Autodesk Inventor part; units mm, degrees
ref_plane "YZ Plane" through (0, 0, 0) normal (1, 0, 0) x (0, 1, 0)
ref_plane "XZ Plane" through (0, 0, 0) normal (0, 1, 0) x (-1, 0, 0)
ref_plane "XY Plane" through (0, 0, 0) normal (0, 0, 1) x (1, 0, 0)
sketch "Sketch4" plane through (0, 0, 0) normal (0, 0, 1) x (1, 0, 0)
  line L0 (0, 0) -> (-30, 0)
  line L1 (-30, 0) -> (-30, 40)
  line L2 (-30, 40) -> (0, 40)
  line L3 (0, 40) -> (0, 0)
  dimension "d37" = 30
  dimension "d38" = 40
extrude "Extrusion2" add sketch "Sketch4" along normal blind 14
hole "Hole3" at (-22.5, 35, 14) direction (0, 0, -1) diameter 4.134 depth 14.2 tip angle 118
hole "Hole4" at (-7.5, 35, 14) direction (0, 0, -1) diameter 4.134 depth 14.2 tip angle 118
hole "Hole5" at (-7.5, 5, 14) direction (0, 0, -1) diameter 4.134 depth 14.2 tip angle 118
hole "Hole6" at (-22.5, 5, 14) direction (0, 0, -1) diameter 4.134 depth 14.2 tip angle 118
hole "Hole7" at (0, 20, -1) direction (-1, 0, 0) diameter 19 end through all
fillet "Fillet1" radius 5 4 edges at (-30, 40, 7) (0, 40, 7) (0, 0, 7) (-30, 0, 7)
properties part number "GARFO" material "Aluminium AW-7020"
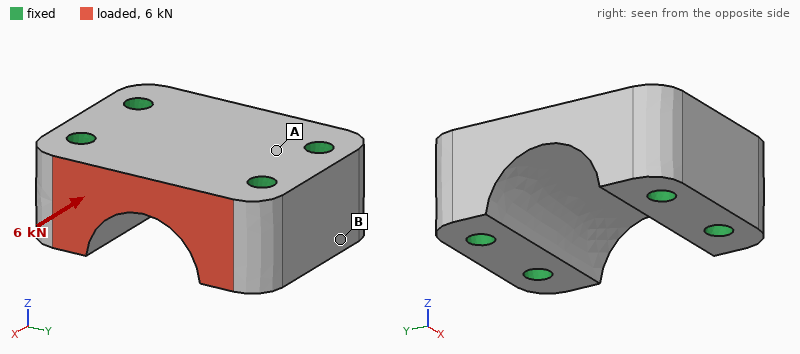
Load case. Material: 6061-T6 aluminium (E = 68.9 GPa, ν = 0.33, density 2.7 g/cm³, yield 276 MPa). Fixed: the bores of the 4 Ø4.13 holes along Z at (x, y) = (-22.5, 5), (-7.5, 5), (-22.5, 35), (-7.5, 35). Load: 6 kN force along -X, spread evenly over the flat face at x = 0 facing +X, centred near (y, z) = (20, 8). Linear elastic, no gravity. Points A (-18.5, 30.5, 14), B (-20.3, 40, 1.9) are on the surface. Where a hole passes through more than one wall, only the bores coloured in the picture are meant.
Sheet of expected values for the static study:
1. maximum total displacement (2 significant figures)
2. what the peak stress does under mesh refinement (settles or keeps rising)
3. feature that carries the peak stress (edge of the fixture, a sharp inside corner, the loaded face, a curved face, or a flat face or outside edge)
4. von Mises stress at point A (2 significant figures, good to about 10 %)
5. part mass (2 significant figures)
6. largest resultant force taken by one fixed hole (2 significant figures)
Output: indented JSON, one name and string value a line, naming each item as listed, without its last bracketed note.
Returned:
{
  "maximum total displacement": "7.0 µm",
  "what the peak stress does under mesh refinement": "keeps rising",
  "feature that carries the peak stress": "edge of the fixture",
  "von Mises stress at point A": "14 MPa",
  "part mass": "33 g",
  "largest resultant force taken by one fixed hole": "2.2 kN"
}
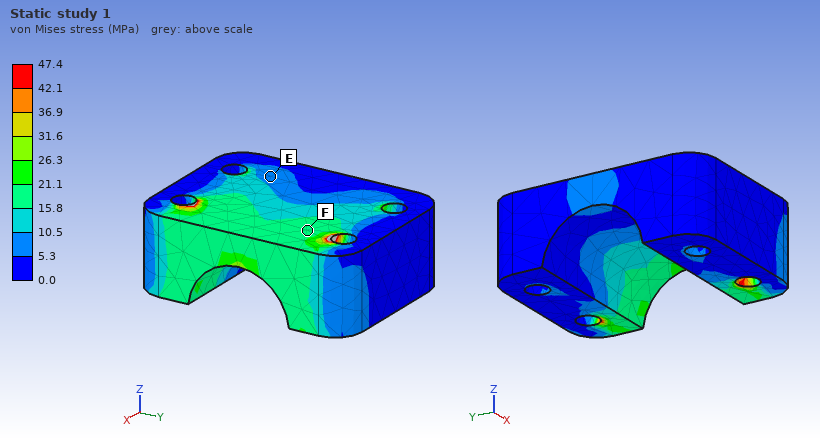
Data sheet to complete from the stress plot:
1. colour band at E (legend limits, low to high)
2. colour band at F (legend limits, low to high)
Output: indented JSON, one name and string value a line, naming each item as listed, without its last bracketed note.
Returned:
{
  "colour band at E": "5.3 to 10.5 MPa",
  "colour band at F": "15.8 to 21.1 MPa"
}
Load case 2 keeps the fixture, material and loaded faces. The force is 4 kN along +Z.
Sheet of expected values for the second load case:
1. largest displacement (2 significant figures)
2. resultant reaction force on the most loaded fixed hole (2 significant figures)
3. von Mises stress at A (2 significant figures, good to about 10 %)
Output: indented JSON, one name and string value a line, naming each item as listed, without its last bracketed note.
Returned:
{
  "largest displacement": "16 µm",
  "resultant reaction force on the most loaded fixed hole": "2.1 kN",
  "von Mises stress at A": "7.5 MPa"
}
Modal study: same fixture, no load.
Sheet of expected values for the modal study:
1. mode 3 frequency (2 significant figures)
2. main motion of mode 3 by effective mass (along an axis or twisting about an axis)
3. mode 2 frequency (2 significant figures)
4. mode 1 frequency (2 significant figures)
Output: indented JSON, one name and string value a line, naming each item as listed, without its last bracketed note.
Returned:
{
  "mode 3 frequency": "58 kHz",
  "main motion of mode 3 by effective mass": "along X",
  "mode 2 frequency": "48 kHz",
  "mode 1 frequency": "48 kHz"
}
